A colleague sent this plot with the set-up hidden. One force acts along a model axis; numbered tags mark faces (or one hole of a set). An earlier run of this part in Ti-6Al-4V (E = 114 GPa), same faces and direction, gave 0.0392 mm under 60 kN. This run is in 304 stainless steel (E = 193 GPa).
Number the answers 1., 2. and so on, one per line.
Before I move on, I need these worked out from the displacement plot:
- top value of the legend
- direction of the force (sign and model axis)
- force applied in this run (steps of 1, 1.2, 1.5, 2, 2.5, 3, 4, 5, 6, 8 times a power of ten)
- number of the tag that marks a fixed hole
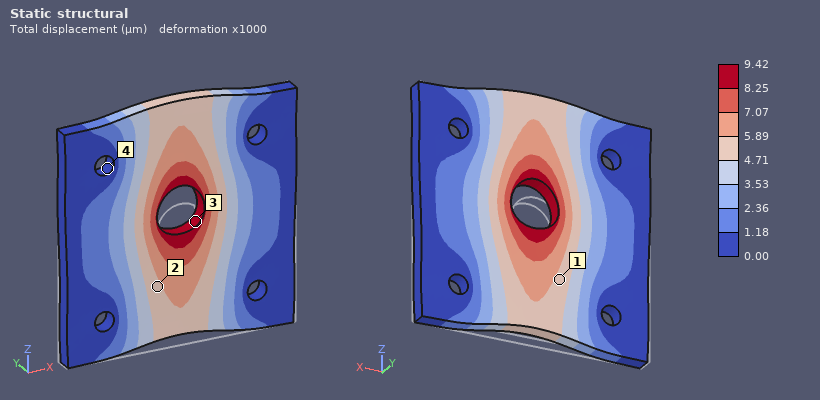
1. 9.42 µm
2. +Z
3. 25 kN
4. 4
